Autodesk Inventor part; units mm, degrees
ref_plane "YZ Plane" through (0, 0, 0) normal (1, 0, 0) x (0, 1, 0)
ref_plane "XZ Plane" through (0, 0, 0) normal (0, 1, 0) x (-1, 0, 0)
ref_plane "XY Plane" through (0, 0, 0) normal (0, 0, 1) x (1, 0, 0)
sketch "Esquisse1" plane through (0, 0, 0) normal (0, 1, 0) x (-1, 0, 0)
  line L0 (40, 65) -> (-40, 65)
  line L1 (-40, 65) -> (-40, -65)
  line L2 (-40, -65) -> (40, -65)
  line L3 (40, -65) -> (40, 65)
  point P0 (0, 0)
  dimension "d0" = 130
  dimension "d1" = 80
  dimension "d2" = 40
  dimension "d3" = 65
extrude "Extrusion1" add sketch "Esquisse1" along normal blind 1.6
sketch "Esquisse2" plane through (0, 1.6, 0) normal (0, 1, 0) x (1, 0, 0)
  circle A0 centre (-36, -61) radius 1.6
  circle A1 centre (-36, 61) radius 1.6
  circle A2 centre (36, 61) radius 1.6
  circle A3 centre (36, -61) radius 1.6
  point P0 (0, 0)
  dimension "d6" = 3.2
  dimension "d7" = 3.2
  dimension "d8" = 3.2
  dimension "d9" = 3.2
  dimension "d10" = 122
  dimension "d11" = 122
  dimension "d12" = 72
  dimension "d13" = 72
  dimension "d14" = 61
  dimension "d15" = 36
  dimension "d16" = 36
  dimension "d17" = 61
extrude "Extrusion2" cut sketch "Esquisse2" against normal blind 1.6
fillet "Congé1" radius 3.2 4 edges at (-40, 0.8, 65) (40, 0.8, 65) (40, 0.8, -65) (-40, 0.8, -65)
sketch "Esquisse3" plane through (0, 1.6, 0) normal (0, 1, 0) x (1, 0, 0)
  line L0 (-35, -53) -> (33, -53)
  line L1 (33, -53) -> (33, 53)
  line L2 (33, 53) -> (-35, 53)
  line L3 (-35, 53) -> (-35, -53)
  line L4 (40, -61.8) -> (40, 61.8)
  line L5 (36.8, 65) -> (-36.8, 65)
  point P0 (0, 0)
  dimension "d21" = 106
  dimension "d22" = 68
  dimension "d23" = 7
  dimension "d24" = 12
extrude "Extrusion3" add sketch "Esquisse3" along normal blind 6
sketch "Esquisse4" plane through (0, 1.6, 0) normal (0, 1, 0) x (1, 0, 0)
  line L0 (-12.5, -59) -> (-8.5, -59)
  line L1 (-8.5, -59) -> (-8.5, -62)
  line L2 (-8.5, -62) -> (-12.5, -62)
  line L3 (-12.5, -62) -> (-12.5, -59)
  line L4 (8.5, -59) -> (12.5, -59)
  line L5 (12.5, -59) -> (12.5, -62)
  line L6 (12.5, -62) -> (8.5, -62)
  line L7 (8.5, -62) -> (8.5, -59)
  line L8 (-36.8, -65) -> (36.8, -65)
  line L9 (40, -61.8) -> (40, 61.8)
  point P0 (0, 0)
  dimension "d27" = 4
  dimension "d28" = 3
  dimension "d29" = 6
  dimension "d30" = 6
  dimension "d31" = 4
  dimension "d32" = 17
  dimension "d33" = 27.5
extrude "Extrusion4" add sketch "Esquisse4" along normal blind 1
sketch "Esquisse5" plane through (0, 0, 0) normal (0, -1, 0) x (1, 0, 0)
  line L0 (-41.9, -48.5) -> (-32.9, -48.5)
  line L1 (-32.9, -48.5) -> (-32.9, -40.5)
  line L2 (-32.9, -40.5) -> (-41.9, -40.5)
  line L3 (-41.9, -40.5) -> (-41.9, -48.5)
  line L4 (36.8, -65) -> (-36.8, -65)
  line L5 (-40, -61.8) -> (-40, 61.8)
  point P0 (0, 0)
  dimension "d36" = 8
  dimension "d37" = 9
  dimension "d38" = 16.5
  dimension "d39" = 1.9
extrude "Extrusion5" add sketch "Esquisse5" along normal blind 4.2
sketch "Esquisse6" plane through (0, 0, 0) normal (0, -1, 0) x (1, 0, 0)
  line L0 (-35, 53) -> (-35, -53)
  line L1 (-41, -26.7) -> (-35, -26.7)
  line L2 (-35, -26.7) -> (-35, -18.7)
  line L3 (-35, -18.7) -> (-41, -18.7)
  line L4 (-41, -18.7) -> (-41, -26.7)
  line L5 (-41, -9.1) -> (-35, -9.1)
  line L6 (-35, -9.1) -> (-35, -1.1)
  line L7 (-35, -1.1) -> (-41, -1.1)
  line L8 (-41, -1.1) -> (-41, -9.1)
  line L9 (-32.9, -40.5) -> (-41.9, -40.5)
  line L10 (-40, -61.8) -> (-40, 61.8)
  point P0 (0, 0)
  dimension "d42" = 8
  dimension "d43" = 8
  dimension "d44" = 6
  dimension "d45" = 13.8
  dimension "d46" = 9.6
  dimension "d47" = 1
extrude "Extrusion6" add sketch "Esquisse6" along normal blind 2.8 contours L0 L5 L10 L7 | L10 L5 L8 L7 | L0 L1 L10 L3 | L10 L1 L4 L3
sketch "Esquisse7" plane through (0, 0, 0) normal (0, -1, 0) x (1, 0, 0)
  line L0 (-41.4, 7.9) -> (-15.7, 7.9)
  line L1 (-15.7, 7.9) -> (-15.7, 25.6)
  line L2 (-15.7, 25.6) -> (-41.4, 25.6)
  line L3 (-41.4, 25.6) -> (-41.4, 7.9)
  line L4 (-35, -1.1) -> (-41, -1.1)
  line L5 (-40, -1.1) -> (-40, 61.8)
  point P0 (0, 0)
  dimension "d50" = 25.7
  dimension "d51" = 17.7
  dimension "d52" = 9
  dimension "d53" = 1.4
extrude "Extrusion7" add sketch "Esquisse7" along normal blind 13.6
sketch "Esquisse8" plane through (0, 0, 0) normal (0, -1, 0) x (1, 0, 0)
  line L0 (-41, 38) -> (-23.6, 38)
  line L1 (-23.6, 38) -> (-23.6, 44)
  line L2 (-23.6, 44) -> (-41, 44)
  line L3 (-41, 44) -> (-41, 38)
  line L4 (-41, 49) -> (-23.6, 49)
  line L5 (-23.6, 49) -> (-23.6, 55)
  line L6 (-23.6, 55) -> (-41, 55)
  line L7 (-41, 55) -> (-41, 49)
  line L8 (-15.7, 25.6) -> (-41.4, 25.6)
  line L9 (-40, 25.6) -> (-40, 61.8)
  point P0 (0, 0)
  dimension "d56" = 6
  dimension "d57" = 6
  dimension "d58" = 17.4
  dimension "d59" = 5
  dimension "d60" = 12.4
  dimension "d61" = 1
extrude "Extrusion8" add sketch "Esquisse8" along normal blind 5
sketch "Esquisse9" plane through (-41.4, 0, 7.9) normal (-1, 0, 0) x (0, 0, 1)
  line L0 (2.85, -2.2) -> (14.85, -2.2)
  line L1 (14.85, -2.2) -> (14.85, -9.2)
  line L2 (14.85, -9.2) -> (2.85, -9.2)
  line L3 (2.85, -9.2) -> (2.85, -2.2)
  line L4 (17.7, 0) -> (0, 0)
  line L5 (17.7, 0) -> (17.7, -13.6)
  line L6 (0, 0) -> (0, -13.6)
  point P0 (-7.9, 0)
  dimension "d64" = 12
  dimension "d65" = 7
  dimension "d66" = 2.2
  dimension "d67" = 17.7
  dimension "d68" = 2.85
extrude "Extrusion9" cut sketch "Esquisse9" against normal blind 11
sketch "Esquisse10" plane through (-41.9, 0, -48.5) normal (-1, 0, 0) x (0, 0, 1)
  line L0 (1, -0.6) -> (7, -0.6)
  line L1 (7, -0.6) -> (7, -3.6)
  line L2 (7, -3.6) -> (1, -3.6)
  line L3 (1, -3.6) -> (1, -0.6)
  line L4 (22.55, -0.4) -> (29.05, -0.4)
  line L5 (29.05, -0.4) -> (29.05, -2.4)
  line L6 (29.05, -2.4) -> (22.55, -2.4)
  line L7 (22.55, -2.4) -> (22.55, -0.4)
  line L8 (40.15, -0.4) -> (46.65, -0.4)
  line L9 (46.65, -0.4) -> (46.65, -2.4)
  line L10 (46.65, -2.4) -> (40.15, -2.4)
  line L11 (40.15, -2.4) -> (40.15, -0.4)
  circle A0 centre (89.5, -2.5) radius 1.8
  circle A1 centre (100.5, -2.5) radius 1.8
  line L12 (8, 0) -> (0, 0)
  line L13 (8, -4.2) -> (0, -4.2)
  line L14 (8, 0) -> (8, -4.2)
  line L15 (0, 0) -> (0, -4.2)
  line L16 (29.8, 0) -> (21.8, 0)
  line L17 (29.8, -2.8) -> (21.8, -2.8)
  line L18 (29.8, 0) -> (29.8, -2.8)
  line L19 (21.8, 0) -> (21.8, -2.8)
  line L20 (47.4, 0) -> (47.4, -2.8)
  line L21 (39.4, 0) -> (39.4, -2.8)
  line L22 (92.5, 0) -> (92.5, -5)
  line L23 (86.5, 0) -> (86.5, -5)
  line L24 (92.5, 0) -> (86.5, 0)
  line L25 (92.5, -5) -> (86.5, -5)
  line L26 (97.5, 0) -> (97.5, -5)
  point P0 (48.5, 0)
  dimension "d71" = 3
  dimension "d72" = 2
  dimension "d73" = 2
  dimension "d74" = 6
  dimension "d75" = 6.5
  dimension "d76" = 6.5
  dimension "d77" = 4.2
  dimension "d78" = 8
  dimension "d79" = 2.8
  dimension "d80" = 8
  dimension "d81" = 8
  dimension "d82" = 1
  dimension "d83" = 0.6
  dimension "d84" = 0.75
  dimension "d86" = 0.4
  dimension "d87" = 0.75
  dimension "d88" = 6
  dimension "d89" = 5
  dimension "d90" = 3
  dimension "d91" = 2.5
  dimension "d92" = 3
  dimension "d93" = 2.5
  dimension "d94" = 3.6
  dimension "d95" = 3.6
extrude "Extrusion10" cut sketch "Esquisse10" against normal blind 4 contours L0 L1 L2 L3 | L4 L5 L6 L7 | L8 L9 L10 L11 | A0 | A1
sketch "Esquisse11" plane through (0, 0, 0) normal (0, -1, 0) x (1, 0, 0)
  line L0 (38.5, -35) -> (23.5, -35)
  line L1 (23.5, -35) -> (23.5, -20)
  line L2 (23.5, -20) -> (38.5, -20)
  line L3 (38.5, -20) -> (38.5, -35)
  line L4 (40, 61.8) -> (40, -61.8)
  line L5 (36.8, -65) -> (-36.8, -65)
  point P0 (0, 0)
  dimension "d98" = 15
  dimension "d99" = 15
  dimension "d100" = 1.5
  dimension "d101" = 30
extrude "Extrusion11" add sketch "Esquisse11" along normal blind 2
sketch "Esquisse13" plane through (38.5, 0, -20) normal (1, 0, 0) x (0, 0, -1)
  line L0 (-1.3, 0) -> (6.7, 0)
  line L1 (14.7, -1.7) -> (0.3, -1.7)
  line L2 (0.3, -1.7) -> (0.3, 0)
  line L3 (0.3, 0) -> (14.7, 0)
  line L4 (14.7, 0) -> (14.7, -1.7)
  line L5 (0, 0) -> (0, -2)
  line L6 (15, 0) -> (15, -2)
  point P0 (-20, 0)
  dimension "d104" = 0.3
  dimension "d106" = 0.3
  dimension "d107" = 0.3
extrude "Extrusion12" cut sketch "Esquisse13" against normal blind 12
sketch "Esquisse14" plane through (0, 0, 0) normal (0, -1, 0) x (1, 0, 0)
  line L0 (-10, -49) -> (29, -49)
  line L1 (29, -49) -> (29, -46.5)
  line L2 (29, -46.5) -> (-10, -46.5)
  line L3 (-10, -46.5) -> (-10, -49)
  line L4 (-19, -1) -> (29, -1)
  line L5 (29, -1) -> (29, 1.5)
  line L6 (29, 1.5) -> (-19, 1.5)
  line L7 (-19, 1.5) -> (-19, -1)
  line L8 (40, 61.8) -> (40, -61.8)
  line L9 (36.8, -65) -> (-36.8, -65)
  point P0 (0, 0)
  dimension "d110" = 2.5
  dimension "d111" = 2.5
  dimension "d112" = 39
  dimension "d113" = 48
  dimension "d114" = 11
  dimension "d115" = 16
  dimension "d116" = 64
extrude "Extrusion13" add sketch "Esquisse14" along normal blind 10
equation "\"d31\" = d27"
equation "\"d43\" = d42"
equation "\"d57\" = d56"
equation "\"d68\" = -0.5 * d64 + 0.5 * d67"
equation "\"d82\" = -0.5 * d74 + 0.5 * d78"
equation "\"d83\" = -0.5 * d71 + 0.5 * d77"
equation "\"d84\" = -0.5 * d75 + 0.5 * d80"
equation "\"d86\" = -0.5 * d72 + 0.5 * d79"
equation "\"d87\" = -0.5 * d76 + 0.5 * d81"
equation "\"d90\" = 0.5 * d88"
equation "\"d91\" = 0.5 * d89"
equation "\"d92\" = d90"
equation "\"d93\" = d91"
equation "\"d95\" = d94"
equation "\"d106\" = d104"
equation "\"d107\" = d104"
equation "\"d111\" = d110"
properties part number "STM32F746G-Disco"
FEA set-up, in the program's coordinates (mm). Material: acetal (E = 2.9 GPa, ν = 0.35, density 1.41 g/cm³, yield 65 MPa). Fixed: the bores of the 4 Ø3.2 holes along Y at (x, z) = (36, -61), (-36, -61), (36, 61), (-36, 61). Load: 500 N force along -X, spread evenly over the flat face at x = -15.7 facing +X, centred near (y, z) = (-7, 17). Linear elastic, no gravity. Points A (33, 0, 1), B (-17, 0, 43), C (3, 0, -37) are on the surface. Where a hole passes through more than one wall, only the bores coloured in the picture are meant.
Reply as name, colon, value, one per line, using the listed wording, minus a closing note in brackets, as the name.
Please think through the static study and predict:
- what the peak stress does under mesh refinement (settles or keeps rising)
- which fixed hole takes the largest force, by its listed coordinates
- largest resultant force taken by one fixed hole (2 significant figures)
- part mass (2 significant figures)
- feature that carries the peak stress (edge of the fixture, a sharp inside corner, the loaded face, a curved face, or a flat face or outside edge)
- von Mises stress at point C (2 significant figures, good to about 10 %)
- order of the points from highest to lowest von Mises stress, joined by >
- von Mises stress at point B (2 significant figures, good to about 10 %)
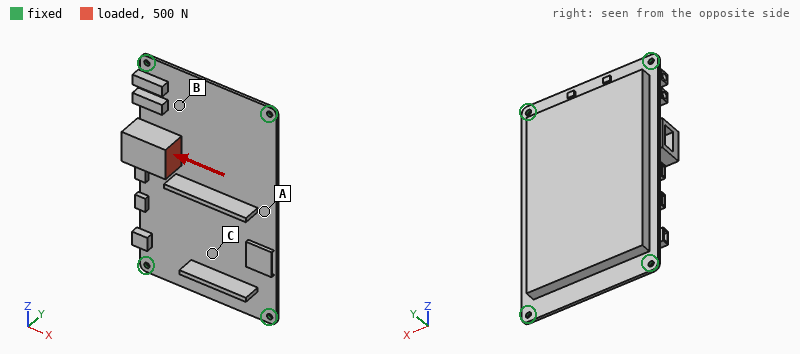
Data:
what the peak stress does under mesh refinement: keeps rising
which fixed hole takes the largest force, by its listed coordinates: (-36, 61)
largest resultant force taken by one fixed hole: 180 N
part mass: 97 g
feature that carries the peak stress: edge of the fixture
von Mises stress at point C: 3.6 MPa
order of the points from highest to lowest von Mises stress, joined by >: B > C > A
von Mises stress at point B: 6.3 MPa
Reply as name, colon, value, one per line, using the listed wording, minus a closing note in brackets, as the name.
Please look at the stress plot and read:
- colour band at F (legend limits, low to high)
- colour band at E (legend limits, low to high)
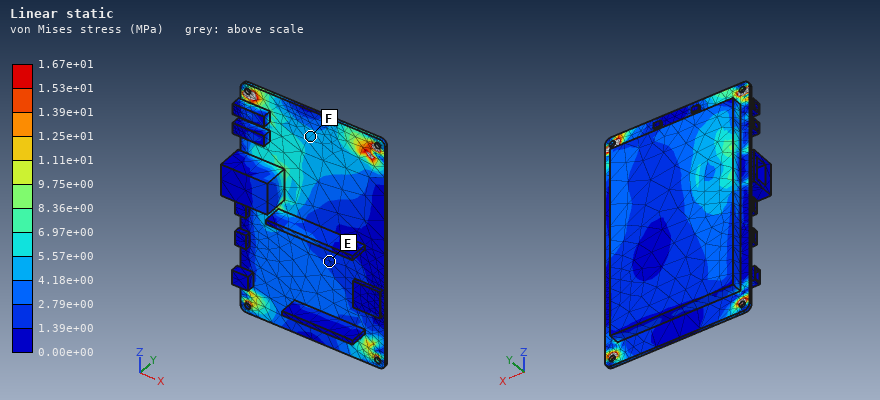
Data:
colour band at F: 4.18e+00 to 5.57e+00 MPa
colour band at E: 1.39e+00 to 2.79e+00 MPa
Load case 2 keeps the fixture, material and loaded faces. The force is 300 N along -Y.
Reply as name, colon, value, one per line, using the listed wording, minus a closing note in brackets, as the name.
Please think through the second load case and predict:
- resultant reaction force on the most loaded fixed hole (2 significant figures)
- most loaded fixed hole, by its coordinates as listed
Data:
resultant reaction force on the most loaded fixed hole: 250 N
most loaded fixed hole, by its coordinates as listed: (-36, 61)
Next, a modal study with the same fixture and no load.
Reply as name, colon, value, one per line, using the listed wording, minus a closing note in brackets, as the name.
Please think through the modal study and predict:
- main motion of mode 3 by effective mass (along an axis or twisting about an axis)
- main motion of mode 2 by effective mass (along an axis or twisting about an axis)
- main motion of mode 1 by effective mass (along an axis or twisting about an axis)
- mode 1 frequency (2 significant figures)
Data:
main motion of mode 3 by effective mass: twisting about X
main motion of mode 2 by effective mass: twisting about Z
main motion of mode 1 by effective mass: along Y
mode 1 frequency: 310 Hz
